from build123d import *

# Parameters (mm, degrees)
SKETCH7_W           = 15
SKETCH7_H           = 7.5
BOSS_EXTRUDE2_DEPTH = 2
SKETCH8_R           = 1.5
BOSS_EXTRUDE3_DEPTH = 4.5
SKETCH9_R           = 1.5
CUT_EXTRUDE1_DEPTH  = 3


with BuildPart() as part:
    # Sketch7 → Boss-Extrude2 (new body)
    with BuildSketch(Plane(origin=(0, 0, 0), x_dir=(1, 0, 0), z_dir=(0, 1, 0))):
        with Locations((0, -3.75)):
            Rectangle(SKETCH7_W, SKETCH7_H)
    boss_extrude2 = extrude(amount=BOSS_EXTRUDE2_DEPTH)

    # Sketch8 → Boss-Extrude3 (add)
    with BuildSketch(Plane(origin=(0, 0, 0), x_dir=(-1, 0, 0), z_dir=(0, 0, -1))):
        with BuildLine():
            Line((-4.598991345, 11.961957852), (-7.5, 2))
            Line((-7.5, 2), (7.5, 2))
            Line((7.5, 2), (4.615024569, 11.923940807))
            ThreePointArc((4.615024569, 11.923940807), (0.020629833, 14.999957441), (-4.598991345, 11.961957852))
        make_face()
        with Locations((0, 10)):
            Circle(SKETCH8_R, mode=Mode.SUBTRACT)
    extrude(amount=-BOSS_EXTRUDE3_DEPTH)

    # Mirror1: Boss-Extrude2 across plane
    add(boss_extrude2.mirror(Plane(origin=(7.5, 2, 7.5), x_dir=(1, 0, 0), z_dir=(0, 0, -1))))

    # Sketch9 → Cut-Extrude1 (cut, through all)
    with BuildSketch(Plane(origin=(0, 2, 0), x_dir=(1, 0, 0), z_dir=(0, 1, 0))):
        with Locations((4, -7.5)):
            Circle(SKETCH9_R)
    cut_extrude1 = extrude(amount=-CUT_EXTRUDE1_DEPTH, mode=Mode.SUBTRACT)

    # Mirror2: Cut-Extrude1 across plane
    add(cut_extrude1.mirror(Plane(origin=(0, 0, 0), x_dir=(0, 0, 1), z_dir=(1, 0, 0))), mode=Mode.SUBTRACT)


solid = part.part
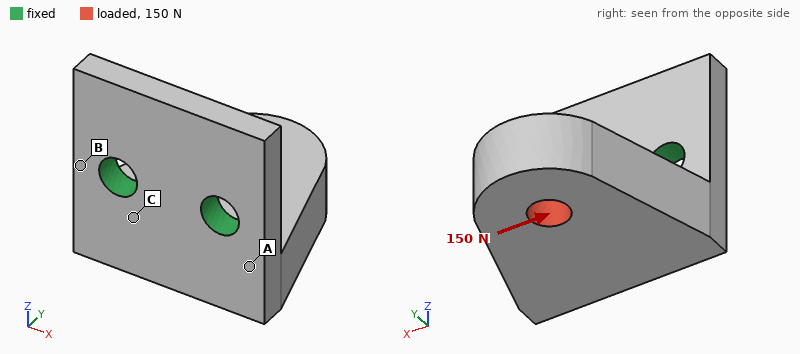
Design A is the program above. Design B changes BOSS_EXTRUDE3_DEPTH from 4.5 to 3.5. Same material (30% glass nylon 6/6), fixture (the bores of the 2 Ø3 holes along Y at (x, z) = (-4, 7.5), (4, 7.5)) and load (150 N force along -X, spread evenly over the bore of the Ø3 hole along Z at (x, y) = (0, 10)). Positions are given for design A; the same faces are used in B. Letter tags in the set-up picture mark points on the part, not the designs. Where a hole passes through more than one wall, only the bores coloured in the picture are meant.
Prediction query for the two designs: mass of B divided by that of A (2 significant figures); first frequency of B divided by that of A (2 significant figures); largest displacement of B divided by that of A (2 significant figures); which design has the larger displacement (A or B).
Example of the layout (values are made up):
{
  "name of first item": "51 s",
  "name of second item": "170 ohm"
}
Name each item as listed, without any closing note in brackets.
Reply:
{
  "mass of B divided by that of A": "0.87",
  "first frequency of B divided by that of A": "0.98",
  "largest displacement of B divided by that of A": "1.6",
  "which design has the larger displacement": "B"
}
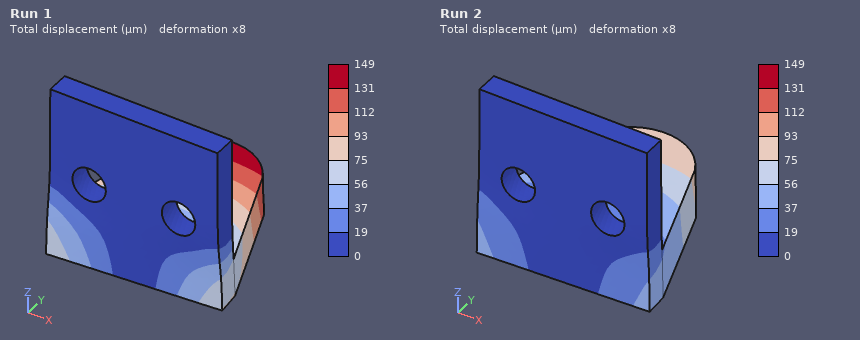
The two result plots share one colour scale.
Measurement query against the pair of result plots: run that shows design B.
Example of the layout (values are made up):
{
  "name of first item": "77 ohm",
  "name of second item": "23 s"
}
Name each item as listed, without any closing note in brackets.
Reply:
{
  "run that shows design B": "Run 1"
}
